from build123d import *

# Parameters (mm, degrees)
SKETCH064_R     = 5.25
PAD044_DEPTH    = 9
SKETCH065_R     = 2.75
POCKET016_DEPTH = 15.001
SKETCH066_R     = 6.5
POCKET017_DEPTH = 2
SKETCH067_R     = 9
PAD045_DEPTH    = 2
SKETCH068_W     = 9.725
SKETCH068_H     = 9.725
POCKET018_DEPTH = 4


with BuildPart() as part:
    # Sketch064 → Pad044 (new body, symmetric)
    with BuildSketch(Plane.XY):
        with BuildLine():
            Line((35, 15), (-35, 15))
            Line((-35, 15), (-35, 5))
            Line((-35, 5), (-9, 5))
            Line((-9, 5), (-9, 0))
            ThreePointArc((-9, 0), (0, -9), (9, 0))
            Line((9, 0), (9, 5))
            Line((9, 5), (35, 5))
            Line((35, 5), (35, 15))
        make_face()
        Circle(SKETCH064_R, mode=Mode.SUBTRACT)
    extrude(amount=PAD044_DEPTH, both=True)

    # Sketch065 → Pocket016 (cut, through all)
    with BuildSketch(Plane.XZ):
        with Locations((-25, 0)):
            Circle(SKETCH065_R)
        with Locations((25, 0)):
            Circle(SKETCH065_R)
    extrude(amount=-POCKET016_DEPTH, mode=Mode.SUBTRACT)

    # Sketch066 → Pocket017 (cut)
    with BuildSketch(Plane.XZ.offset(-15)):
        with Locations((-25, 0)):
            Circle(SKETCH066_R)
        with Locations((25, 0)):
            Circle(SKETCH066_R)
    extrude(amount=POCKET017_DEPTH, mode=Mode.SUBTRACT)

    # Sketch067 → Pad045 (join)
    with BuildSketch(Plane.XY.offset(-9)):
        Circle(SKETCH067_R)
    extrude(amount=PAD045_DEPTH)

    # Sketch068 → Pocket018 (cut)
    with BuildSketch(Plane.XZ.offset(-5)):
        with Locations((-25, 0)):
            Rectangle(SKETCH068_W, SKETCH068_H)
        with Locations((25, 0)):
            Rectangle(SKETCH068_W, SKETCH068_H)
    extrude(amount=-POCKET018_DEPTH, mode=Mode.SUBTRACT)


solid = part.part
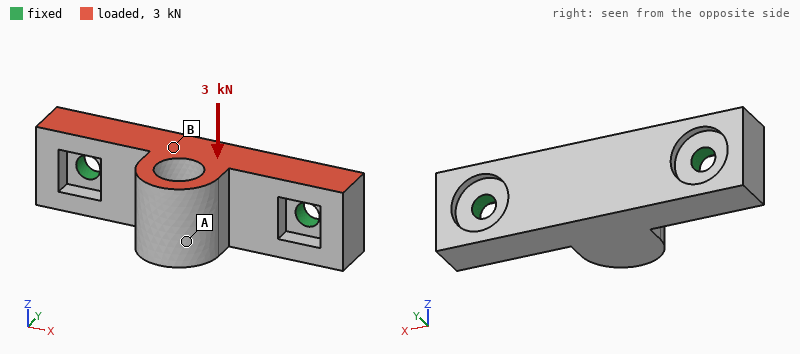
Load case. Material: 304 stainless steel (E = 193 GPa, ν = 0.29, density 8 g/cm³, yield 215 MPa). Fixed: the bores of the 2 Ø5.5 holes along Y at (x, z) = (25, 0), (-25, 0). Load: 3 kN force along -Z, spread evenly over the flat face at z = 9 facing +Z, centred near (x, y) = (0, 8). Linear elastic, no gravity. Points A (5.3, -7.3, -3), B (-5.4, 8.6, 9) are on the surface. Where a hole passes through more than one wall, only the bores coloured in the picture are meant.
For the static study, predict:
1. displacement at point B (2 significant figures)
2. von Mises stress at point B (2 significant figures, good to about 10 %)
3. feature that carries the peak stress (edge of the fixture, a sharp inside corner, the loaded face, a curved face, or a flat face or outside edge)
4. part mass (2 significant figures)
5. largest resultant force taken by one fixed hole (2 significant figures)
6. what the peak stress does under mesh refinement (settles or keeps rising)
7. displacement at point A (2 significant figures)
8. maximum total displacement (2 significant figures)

6.3 µm
18 MPa
edge of the fixture
110 g
1.5 kN
keeps rising
13 µm
15 µm
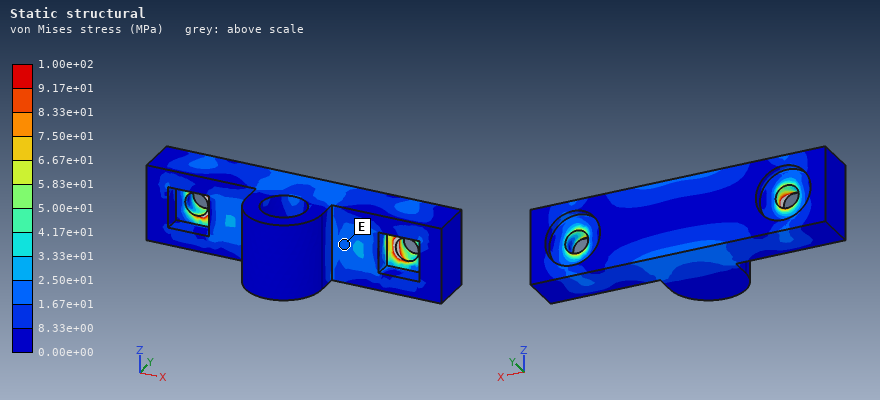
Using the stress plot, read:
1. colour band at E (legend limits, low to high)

1.67e+01 to 2.50e+01 MPa
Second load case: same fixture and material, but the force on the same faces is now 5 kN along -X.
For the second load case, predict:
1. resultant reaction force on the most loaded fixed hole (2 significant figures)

2.6 kN
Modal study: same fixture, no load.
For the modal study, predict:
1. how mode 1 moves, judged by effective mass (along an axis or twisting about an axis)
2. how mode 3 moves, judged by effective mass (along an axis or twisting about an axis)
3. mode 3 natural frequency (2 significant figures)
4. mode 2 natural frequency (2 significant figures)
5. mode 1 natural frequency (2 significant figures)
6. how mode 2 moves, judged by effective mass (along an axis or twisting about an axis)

along Z
along Z
16 kHz
10 kHz
7600 Hz
along Y
